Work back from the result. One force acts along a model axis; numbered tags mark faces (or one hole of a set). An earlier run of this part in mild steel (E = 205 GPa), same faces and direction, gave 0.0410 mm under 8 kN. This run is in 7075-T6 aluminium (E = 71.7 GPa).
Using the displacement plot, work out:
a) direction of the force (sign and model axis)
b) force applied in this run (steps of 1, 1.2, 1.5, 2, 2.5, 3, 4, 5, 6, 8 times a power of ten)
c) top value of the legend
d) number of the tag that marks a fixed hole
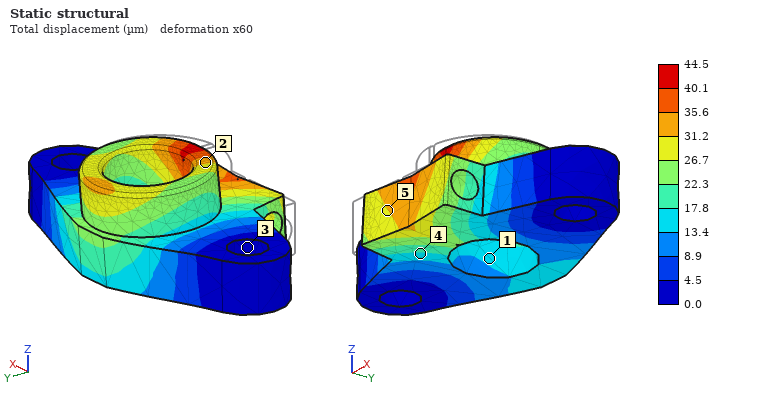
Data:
+Y
3 kN
44.5 µm
3
